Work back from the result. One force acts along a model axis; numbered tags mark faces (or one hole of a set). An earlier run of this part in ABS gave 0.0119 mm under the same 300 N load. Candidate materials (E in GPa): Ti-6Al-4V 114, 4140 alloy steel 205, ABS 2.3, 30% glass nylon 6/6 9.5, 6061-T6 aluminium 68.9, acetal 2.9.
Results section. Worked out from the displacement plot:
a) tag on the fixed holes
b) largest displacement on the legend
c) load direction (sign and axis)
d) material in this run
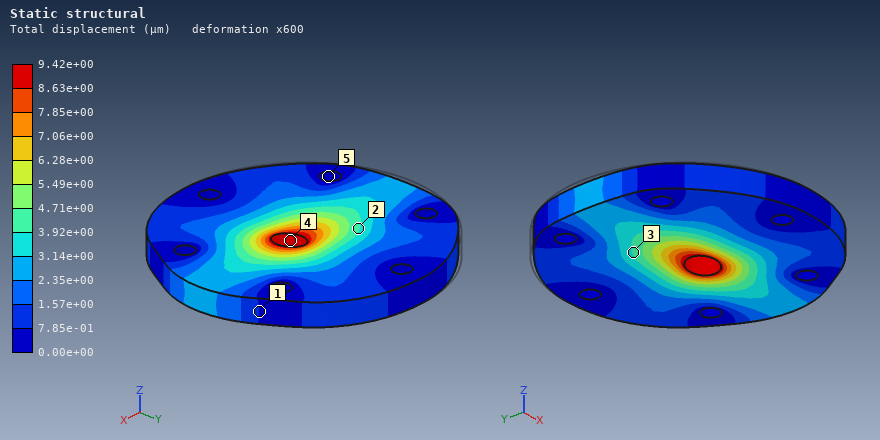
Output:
5
9.42e+00 µm
+X
acetal
